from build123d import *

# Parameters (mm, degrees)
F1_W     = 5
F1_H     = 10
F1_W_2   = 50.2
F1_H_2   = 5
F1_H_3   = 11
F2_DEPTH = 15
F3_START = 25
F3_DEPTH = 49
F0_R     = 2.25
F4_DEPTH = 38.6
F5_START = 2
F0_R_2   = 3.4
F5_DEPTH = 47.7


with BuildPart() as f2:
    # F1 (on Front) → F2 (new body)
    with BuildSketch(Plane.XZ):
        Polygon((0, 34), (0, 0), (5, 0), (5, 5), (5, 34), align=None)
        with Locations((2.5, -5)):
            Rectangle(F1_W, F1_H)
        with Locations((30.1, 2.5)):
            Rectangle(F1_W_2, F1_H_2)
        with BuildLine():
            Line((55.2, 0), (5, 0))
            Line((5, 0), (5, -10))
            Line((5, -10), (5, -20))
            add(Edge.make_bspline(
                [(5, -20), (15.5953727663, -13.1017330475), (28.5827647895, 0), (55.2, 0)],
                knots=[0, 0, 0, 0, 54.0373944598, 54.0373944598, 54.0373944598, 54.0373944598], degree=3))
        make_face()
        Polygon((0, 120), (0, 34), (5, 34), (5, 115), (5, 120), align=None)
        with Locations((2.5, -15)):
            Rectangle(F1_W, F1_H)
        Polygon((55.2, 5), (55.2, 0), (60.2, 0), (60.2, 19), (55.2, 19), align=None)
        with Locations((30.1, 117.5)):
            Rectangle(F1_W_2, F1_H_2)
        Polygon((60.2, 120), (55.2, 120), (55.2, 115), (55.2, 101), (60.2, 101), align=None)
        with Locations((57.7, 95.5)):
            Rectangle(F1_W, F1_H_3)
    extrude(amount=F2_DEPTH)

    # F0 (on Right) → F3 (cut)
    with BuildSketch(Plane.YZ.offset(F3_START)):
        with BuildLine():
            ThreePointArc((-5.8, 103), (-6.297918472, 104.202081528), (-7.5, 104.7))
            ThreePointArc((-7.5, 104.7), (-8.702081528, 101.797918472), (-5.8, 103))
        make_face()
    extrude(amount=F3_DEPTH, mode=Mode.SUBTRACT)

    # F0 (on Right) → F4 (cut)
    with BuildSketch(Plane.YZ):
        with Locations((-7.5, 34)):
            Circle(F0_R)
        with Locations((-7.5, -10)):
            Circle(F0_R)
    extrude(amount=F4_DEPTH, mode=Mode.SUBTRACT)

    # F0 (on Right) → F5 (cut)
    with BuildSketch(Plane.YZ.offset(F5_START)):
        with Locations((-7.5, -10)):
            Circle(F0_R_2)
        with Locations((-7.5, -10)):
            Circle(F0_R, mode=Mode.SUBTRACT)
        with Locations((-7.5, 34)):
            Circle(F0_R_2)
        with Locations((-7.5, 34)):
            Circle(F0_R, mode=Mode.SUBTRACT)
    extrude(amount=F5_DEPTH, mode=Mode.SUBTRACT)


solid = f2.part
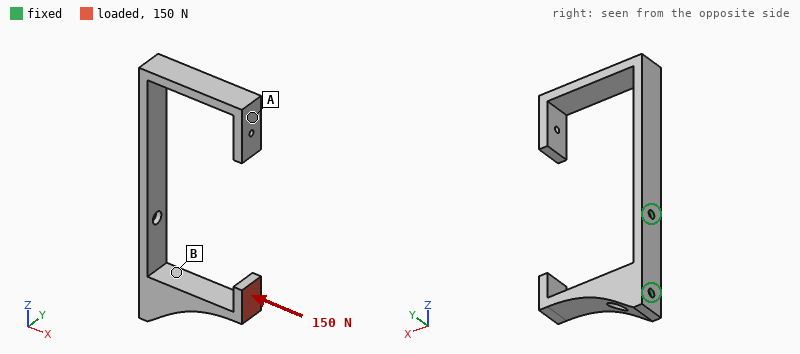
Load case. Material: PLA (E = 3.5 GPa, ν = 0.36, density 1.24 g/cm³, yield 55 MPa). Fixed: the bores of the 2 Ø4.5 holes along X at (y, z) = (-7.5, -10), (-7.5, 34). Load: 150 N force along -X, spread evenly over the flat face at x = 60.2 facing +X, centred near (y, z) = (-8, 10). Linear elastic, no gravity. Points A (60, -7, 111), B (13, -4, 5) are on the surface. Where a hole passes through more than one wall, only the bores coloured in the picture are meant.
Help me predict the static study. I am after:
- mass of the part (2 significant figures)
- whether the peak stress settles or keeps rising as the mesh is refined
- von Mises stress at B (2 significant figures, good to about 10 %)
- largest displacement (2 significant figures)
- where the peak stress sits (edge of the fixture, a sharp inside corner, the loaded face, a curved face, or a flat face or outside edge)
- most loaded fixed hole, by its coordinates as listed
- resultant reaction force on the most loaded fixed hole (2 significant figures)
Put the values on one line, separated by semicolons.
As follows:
32 g; keeps rising; 3.4 MPa; 1.6 mm; edge of the fixture; (-7.5, -10); 170 N
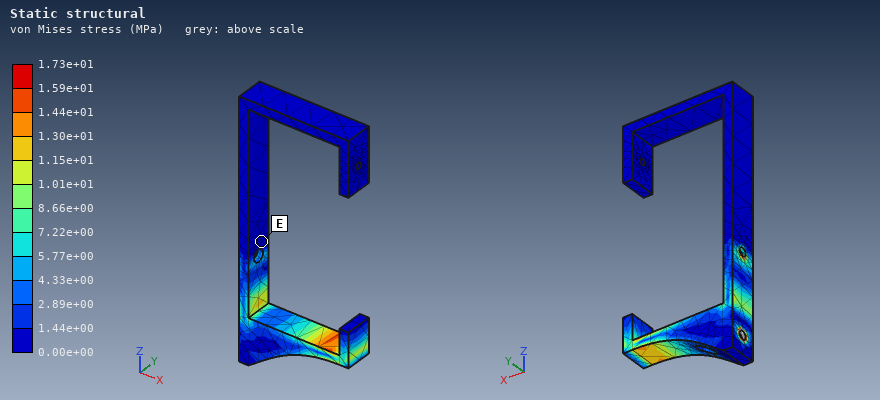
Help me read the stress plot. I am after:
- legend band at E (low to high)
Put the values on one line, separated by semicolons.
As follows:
0.00e+00 to 1.44e+00 MPa
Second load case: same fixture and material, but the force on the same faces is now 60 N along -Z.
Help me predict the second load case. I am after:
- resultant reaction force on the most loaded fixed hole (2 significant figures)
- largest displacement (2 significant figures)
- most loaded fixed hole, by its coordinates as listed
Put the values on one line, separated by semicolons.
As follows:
190 N; 1.6 mm; (-7.5, 34)
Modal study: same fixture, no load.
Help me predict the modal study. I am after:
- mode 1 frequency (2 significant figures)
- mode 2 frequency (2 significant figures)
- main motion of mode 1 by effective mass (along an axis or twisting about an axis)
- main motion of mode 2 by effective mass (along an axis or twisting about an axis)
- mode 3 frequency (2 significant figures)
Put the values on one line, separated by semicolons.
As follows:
69 Hz; 110 Hz; along X; along Y; 190 Hz
